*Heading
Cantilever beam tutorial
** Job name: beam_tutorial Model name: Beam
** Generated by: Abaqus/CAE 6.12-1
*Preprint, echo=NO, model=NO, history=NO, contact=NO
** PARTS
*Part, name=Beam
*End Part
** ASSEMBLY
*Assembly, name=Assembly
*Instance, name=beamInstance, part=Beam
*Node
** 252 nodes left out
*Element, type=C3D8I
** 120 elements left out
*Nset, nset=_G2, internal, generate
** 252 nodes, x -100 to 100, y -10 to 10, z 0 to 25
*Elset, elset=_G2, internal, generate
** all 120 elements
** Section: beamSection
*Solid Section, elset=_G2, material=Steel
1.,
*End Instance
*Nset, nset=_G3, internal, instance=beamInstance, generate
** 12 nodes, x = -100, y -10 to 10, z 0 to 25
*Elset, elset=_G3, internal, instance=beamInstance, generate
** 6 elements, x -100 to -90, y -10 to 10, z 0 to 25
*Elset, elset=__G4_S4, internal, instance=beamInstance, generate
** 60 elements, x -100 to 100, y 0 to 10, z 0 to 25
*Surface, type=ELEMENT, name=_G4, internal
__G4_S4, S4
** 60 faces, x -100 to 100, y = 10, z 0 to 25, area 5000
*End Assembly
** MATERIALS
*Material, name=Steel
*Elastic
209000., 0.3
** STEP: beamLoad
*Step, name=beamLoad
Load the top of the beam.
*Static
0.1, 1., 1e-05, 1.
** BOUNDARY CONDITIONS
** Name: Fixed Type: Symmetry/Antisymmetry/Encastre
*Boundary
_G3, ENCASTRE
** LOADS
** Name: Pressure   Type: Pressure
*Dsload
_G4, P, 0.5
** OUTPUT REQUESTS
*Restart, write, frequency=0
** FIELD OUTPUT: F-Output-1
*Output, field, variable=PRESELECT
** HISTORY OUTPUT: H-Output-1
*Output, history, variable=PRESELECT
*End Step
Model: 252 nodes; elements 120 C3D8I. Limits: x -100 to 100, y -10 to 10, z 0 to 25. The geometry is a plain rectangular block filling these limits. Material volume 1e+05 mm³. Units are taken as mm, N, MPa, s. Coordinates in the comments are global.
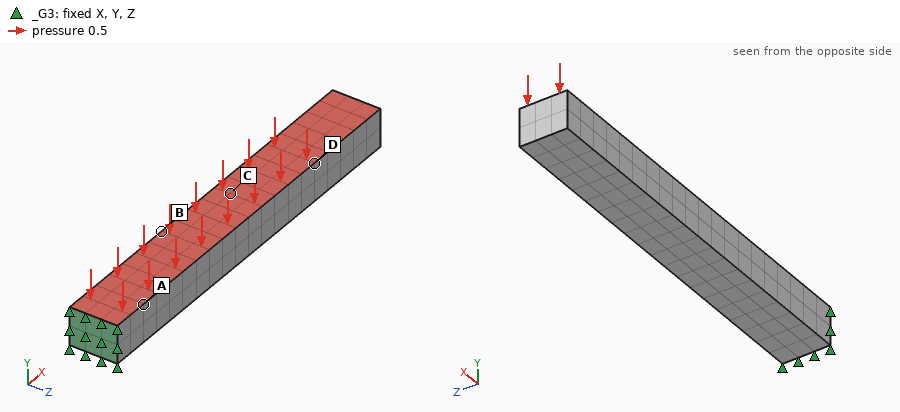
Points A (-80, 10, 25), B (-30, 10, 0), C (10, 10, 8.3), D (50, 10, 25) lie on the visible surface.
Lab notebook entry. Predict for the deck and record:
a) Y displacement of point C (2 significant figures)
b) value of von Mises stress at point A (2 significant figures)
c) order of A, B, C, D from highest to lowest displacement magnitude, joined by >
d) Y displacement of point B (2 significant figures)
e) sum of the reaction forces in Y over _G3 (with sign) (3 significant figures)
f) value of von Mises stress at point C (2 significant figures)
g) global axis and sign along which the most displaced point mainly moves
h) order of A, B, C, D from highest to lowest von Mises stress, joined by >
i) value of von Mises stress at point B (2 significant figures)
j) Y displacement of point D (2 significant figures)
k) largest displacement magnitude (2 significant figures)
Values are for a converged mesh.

-0.30 mm
120 MPa
D > C > B > A
-0.14 mm
2500 N
31 MPa
-Y
A > B > C > D
64 MPa
-0.48 mm
0.72 mm
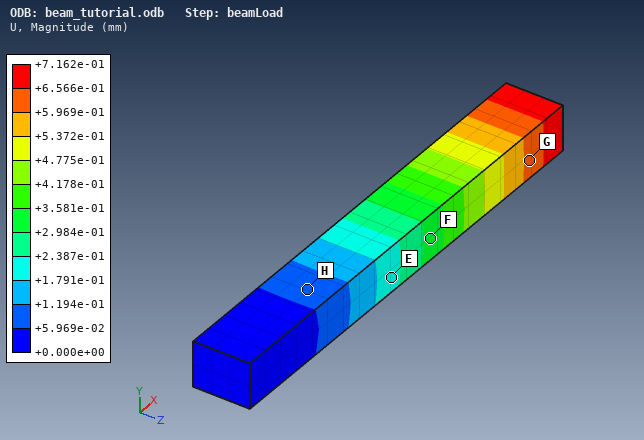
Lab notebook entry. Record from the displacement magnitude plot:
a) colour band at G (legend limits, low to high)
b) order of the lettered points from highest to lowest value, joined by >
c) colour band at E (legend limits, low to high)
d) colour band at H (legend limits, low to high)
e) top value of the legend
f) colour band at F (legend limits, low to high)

+5.969e-01 to +6.566e-01 mm
G > F > E > H
+1.791e-01 to +2.387e-01 mm
+5.969e-02 to +1.194e-01 mm
+7.162e-01 mm
+2.984e-01 to +3.581e-01 mm
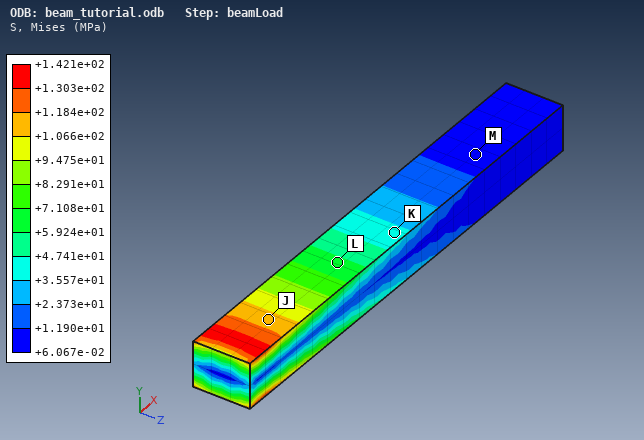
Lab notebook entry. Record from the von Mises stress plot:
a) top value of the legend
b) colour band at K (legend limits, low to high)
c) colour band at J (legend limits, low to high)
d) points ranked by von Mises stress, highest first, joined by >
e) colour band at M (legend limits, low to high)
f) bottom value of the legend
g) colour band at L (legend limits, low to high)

+1.421e+02 MPa
+3.557e+01 to +4.741e+01 MPa
+1.066e+02 to +1.184e+02 MPa
J > L > K > M
+6.067e-02 to +1.190e+01 MPa
+6.067e-02 MPa
+5.924e+01 to +7.108e+01 MPa
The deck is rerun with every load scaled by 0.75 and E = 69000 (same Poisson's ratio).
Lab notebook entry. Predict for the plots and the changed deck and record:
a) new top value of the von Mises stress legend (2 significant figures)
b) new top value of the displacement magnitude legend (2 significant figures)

110 MPa
1.6 mm
